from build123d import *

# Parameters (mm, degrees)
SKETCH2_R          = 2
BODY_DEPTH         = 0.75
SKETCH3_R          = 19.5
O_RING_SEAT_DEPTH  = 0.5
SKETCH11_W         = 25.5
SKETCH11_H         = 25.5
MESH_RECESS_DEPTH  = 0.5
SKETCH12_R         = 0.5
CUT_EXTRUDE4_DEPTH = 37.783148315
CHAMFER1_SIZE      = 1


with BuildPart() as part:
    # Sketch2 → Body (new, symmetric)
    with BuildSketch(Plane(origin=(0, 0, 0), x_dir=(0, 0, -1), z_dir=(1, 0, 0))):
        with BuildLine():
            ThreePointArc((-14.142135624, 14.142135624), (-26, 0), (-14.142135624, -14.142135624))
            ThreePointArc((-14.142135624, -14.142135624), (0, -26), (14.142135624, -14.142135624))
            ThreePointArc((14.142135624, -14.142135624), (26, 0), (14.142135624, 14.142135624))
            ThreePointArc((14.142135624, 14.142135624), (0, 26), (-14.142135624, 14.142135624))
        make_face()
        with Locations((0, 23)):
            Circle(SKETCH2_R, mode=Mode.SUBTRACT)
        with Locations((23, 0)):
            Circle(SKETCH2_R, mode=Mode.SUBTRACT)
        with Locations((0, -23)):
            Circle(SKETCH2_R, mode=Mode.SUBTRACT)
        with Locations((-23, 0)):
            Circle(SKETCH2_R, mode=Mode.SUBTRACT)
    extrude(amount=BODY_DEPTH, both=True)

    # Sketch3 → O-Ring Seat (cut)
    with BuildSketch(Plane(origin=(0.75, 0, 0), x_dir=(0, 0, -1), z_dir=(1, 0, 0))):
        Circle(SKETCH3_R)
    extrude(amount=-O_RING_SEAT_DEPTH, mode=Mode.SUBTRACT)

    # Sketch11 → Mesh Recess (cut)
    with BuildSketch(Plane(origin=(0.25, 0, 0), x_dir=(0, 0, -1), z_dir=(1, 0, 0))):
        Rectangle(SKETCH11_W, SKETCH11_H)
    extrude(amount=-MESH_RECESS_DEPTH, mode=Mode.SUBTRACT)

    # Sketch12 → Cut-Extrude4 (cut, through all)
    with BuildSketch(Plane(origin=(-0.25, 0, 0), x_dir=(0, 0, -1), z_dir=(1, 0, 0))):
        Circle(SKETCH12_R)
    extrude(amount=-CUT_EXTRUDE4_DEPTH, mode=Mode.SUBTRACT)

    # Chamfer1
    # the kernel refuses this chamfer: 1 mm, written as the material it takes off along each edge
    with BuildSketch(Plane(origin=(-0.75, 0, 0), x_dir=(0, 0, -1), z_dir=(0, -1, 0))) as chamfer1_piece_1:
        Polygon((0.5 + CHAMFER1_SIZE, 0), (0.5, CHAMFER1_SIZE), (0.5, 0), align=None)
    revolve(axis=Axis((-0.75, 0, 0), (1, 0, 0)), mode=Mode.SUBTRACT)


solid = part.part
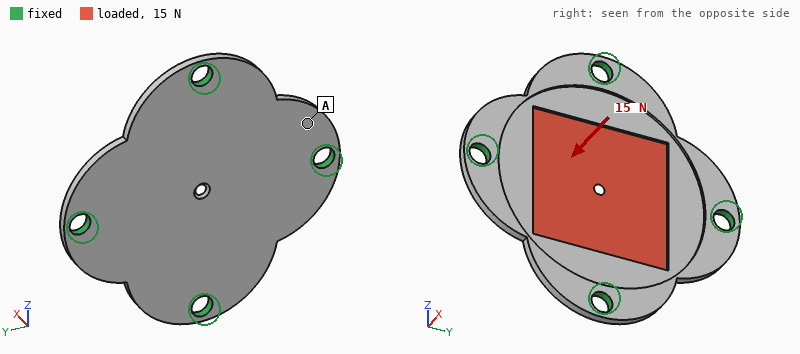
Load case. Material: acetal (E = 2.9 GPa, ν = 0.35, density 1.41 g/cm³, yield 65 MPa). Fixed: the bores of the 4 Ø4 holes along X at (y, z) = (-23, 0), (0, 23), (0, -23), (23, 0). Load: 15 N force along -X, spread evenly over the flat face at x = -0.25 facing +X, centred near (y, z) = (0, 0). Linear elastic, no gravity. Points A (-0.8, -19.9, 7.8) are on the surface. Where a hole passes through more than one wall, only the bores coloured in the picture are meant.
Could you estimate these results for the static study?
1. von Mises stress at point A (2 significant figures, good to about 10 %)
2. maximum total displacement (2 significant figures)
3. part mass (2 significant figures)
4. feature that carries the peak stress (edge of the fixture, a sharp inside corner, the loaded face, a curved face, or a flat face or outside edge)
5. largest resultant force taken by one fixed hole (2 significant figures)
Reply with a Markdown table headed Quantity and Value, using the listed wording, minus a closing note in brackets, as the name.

| Quantity | Value |
|---|---|
| von Mises stress at point A | 2.5 MPa |
| maximum total displacement | 0.73 mm |
| part mass | 2.4 g |
| feature that carries the peak stress | the loaded face |
| largest resultant force taken by one fixed hole | 14 N |
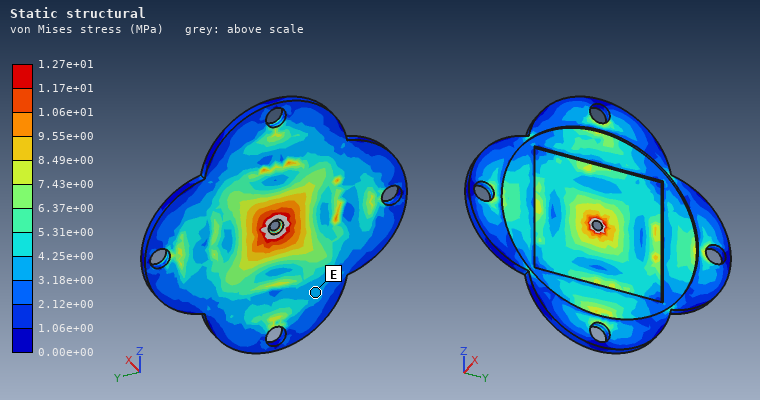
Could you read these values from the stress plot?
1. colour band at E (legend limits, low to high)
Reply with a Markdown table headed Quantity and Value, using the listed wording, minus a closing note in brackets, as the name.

| Quantity | Value |
|---|---|
| colour band at E | 3.18e+00 to 4.25e+00 MPa |
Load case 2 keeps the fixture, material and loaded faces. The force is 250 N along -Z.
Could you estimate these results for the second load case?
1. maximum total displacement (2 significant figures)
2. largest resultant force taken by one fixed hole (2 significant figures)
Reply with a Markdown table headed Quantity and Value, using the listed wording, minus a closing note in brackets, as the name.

| Quantity | Value |
|---|---|
| maximum total displacement | 0.17 mm |
| largest resultant force taken by one fixed hole | 80 N |
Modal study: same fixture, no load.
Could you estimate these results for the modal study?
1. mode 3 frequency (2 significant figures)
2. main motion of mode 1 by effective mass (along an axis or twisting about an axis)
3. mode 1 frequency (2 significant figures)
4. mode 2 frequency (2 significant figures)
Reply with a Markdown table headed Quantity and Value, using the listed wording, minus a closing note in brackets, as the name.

| Quantity | Value |
|---|---|
| mode 3 frequency | 2200 Hz |
| main motion of mode 1 by effective mass | along X |
| mode 1 frequency | 1400 Hz |
| mode 2 frequency | 2200 Hz |
